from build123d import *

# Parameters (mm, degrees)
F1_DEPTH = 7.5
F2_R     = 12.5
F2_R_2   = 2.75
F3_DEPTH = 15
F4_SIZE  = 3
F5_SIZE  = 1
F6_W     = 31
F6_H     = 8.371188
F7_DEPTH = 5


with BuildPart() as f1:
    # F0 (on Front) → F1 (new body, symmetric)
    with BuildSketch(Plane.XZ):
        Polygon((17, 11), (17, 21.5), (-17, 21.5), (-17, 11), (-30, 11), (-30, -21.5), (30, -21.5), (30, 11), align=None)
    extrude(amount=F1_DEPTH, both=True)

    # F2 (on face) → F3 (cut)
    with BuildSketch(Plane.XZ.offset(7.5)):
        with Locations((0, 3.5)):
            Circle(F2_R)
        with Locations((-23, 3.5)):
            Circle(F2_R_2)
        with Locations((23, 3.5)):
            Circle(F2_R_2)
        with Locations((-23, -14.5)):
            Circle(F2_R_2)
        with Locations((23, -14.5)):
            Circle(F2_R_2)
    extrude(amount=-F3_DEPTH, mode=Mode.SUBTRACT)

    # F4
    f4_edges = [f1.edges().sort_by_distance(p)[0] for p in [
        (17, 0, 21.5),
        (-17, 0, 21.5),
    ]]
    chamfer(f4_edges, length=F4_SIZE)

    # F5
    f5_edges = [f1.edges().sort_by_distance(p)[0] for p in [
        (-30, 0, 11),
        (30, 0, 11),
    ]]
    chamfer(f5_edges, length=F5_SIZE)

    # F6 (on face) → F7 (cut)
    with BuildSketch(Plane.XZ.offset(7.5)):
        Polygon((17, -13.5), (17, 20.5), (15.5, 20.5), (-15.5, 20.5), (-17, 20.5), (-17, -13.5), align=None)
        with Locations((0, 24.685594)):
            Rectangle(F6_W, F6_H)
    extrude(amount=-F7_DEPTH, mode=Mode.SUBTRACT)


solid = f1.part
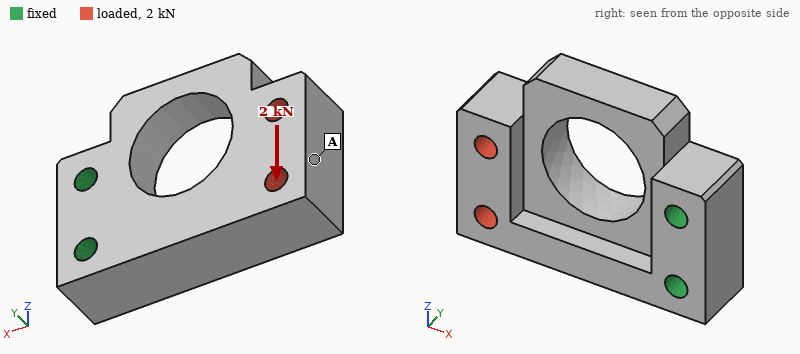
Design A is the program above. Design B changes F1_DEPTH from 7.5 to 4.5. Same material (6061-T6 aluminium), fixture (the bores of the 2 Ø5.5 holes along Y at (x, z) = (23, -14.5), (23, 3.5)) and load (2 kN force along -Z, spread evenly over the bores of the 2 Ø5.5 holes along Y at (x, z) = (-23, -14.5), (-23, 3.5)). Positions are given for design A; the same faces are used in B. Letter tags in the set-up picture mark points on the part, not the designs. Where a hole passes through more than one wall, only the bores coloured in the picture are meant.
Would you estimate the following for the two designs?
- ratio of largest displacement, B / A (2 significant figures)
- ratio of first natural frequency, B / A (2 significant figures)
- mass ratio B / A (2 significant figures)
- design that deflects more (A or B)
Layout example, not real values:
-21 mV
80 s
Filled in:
1.4
0.69
0.63
B
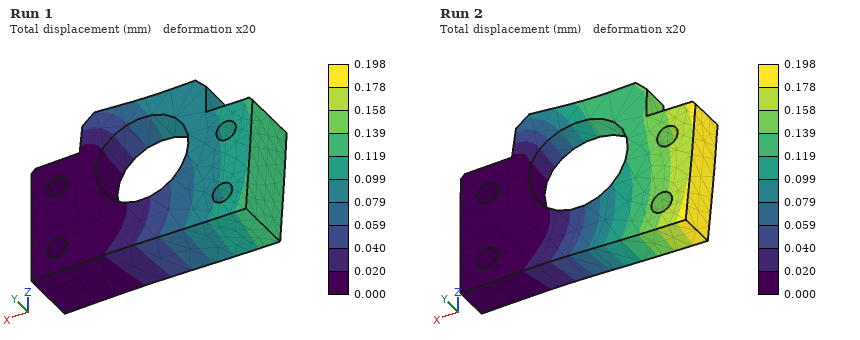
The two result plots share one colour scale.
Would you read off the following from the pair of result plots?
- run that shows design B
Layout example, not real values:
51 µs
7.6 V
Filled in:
Run 2
